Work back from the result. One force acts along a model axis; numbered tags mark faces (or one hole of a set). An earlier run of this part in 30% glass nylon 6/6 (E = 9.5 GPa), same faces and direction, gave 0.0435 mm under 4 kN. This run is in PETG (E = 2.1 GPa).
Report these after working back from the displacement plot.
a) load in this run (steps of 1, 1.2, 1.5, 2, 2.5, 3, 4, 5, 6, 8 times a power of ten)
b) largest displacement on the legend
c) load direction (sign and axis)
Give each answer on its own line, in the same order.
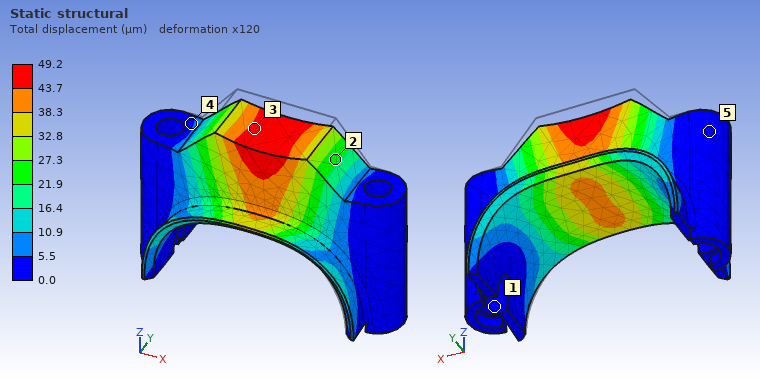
1 kN
49.2 µm
-Z
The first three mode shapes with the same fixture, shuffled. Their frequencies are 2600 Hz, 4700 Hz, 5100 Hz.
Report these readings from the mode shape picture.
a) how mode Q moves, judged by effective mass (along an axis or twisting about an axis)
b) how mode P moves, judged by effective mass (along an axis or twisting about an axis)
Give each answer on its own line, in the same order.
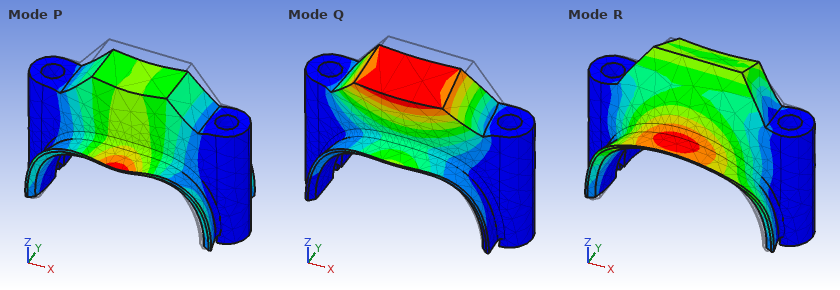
along Y
along Z
